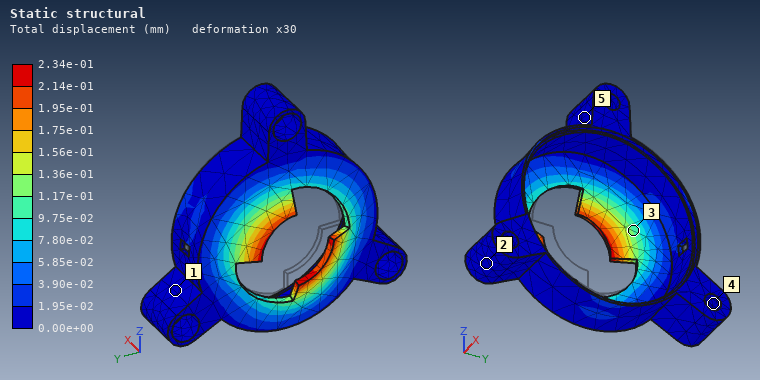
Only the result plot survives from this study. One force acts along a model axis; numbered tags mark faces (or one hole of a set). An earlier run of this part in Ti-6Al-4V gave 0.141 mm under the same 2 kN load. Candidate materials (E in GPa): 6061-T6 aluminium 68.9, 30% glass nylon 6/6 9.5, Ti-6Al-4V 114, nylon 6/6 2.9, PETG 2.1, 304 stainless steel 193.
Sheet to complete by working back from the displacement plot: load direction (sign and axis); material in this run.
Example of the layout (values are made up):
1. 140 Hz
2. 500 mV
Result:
1. -X
2. 6061-T6 aluminium
